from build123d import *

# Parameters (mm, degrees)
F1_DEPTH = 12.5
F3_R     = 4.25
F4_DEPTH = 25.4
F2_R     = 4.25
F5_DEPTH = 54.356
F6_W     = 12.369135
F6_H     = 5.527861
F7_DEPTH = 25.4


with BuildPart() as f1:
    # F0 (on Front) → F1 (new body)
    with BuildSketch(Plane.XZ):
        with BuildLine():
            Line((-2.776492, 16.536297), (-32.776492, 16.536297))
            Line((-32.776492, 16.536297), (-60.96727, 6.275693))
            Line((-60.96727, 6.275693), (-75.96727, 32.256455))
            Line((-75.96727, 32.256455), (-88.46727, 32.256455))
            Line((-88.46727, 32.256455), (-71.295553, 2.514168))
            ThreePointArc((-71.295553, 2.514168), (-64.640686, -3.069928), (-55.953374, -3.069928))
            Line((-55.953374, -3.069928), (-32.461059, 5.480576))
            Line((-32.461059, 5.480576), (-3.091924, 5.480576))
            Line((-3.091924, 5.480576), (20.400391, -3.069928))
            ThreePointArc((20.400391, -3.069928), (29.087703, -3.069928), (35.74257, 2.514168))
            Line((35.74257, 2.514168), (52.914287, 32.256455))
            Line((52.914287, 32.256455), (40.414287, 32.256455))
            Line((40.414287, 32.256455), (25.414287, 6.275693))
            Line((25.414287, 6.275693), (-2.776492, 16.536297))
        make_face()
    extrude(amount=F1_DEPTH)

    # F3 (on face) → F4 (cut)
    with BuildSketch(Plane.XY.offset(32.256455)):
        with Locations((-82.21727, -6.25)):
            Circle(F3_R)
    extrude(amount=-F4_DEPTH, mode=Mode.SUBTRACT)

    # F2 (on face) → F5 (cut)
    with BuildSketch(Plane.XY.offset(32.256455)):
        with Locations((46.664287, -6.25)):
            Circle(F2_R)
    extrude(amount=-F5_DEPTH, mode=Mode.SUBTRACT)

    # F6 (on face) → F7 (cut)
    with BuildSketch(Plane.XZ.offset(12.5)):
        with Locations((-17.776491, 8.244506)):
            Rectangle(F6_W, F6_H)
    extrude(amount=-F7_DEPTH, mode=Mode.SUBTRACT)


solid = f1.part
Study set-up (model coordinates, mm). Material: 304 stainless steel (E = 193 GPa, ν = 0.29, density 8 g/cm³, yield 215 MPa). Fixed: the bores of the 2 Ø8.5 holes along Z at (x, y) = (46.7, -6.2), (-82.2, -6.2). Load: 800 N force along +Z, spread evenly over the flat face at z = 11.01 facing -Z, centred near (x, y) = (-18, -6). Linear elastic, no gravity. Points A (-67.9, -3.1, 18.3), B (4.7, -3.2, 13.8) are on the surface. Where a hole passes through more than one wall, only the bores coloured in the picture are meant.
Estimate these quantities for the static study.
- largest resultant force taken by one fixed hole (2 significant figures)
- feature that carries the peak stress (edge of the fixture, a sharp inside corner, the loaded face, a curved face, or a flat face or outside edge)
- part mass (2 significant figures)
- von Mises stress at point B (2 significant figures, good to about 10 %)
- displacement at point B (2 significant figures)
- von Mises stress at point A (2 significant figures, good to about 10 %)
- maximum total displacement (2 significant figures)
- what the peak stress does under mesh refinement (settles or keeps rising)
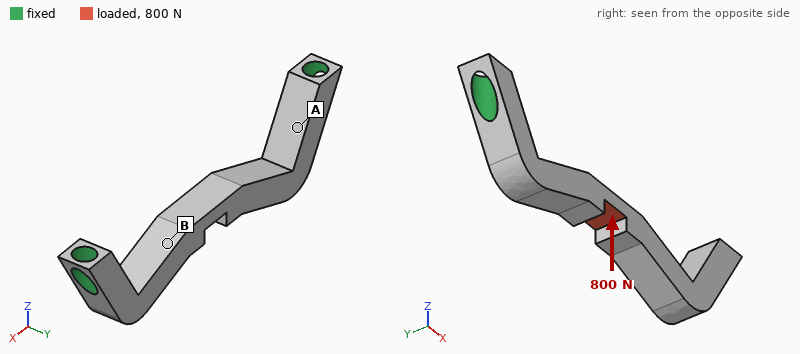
700 N
edge of the fixture
160 g
11 MPa
41 µm
62 MPa
66 µm
keeps rising
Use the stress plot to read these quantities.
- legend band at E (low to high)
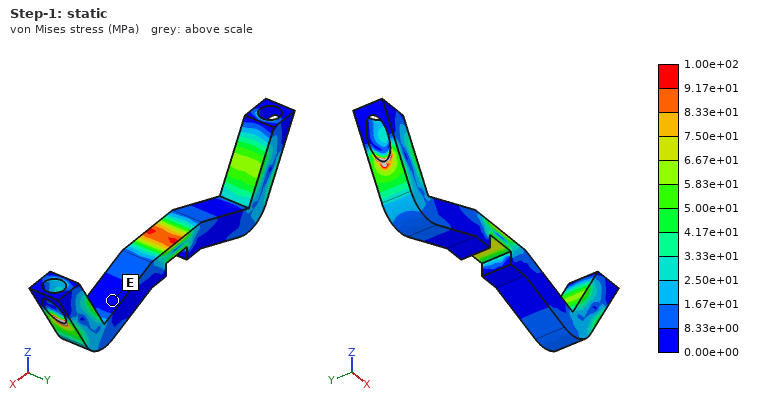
0.00e+00 to 8.33e+00 MPa
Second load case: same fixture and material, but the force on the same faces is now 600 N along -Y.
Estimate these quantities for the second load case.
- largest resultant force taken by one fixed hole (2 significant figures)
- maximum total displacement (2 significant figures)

300 N
40 µm
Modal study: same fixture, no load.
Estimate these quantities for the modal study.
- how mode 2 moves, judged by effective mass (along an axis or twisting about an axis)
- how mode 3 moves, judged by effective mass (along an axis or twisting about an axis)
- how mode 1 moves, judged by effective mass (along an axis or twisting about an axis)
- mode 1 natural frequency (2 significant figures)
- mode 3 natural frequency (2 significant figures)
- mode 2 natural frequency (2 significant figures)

along Y
along X
along Z
2700 Hz
6300 Hz
2900 Hz
